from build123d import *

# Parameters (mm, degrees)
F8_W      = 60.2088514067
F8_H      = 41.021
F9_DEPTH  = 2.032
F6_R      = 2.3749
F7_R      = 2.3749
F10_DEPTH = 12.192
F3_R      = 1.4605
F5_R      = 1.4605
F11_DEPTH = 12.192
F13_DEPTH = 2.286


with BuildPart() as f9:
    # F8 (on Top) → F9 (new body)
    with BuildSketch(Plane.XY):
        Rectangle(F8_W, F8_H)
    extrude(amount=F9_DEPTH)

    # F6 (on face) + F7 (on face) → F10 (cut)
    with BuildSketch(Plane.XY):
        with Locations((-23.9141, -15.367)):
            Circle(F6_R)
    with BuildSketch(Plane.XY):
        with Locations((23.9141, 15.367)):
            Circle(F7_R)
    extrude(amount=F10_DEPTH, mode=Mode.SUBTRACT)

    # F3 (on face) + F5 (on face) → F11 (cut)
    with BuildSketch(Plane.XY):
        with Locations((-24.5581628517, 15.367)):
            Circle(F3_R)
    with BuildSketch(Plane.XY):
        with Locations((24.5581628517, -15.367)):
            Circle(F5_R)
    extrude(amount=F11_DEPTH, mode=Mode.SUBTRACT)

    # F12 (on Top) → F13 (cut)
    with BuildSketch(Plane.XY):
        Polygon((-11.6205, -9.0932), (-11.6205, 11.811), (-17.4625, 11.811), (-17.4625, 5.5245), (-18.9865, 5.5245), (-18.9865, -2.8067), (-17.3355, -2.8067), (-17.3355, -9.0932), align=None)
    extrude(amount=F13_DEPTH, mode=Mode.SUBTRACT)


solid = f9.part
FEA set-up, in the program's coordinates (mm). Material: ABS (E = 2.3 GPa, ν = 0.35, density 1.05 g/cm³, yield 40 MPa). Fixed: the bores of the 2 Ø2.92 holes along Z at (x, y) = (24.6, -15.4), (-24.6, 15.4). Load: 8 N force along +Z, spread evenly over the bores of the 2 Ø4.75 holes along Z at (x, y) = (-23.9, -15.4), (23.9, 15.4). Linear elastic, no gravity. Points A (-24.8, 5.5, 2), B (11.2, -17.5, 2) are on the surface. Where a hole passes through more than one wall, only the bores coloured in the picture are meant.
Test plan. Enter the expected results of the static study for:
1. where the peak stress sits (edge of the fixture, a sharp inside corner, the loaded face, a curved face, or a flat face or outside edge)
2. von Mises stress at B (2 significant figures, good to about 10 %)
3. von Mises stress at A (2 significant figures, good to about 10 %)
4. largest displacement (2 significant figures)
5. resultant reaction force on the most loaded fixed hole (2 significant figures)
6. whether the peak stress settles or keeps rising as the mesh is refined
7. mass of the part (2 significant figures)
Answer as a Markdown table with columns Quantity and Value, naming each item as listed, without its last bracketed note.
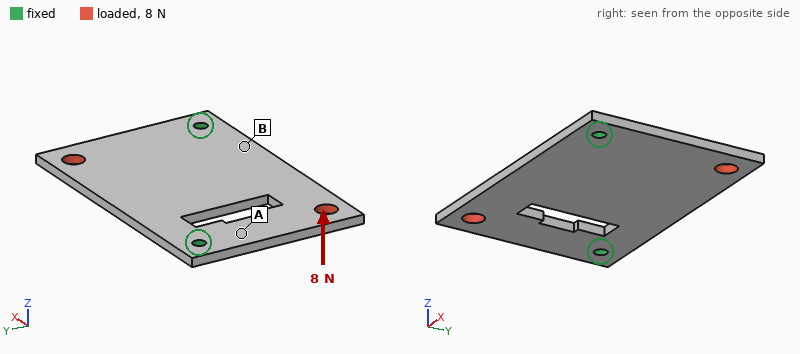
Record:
| Quantity | Value |
|---|---|
| where the peak stress sits | edge of the fixture |
| von Mises stress at B | 1.5 MPa |
| von Mises stress at A | 3.4 MPa |
| largest displacement | 0.77 mm |
| resultant reaction force on the most loaded fixed hole | 4.2 N |
| whether the peak stress settles or keeps rising as the mesh is refined | keeps rising |
| mass of the part | 4.9 g |
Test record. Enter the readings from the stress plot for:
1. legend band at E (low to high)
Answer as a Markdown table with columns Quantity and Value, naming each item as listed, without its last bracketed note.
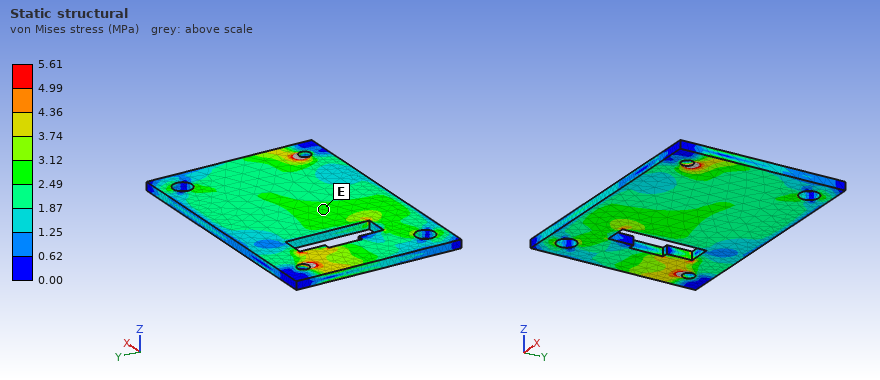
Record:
| Quantity | Value |
|---|---|
| legend band at E | 2.49 to 3.12 MPa |
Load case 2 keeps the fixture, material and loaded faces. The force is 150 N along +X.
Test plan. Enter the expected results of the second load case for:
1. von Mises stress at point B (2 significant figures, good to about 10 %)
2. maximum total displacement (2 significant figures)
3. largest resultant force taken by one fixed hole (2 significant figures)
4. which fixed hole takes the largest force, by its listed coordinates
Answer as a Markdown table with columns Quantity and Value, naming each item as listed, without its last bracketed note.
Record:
| Quantity | Value |
|---|---|
| von Mises stress at point B | 3.4 MPa |
| maximum total displacement | 82 µm |
| largest resultant force taken by one fixed hole | 80 N |
| which fixed hole takes the largest force, by its listed coordinates | (24.6, -15.4) |
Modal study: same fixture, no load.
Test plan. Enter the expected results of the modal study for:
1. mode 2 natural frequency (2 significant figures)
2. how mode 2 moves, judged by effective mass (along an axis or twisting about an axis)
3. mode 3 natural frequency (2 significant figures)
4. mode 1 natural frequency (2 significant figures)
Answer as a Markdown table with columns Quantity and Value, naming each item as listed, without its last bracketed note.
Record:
| Quantity | Value |
|---|---|
| mode 2 natural frequency | 550 Hz |
| how mode 2 moves, judged by effective mass | along Z |
| mode 3 natural frequency | 1100 Hz |
| mode 1 natural frequency | 430 Hz |
